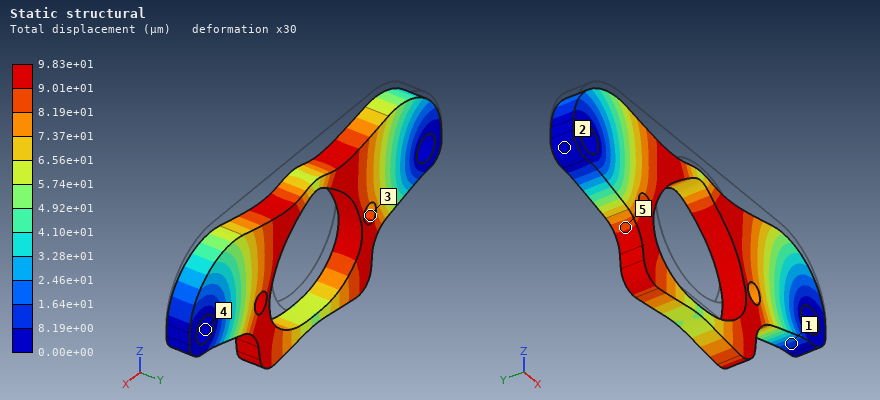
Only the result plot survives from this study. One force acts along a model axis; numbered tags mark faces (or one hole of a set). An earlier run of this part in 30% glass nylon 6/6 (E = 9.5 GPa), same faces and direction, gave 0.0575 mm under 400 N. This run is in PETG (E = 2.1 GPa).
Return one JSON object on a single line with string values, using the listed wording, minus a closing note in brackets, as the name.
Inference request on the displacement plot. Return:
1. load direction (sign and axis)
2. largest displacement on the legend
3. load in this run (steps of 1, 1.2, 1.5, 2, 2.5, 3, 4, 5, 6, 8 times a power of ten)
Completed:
{"load direction": "-Z", "largest displacement on the legend": "9.83e+01 µm", "load in this run": "150 N"}
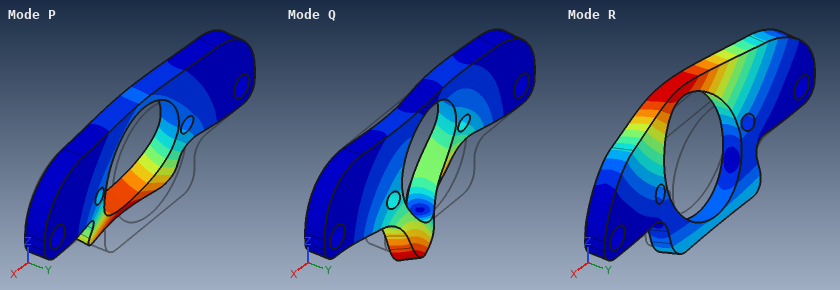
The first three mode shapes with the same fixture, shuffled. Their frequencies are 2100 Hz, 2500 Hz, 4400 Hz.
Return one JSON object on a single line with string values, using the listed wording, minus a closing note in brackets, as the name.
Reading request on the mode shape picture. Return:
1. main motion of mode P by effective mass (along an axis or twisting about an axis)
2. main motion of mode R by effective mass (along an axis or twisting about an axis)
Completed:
{"main motion of mode P by effective mass": "along Y", "main motion of mode R by effective mass": "along Y"}
